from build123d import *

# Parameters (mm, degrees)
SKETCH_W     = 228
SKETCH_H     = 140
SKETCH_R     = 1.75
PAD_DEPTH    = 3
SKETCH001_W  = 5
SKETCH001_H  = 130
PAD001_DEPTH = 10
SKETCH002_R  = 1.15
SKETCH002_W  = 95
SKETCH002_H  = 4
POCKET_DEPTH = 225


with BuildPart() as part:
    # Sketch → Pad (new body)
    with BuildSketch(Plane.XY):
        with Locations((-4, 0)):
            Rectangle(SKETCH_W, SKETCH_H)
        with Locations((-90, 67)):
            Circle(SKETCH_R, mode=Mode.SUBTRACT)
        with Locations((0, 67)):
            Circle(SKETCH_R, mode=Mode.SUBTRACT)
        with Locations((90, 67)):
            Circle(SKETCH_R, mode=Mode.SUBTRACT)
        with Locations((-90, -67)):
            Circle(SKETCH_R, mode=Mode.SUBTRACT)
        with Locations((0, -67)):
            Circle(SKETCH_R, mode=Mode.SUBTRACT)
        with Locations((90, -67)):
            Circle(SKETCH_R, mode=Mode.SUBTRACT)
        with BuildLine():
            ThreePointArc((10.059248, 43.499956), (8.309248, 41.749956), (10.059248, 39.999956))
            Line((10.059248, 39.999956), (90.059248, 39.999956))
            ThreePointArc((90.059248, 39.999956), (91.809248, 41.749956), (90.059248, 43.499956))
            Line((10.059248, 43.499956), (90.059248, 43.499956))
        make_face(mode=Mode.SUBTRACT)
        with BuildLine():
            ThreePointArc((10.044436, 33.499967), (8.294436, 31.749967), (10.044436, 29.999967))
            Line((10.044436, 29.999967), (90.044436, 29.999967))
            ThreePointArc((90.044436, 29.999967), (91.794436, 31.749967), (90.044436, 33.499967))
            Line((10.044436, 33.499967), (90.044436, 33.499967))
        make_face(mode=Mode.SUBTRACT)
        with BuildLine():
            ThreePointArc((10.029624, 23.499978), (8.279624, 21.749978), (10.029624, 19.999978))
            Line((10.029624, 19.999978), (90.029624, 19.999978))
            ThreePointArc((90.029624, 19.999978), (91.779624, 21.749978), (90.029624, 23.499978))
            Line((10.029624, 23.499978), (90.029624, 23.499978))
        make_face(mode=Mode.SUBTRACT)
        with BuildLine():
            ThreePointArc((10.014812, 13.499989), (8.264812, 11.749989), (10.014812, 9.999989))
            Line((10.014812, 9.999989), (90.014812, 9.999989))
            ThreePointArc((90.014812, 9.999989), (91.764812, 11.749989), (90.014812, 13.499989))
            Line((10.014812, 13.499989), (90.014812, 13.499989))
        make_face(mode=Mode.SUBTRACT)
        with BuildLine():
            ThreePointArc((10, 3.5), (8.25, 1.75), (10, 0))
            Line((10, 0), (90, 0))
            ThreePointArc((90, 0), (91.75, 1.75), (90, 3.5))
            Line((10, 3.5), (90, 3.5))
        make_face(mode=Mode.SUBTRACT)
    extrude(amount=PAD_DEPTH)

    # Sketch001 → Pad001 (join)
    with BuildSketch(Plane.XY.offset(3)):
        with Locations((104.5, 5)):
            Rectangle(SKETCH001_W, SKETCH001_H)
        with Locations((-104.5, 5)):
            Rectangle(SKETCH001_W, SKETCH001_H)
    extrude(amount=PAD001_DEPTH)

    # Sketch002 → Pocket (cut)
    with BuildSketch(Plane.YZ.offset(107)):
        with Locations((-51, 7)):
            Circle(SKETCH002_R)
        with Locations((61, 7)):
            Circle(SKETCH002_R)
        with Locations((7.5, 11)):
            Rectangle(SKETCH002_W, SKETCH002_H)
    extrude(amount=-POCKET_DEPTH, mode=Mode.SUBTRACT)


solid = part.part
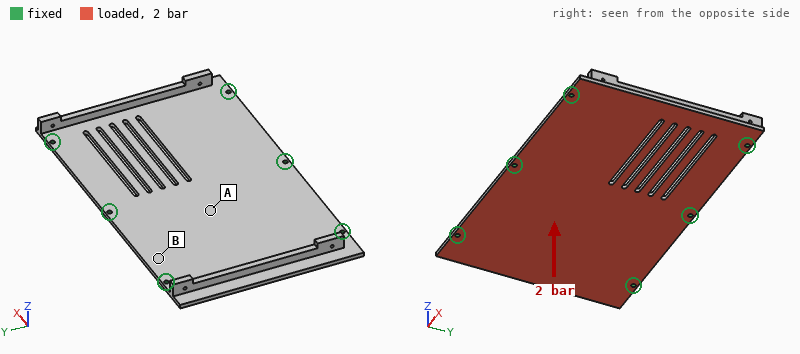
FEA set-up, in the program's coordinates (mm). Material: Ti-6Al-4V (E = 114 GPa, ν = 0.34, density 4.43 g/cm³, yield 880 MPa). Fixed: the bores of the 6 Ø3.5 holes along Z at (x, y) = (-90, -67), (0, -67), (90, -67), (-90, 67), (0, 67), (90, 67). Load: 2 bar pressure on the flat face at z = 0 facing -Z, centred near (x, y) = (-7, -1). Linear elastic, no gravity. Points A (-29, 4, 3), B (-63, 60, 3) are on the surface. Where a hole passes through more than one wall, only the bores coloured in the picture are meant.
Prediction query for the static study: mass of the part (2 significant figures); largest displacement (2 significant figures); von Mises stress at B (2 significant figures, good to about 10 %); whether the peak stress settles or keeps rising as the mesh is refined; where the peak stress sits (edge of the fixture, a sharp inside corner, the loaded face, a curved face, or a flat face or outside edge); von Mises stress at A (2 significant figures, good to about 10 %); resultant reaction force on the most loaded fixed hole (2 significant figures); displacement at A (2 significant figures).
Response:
440 g
1.5 mm
46 MPa
keeps rising
edge of the fixture
120 MPa
1.5 kN
1.1 mm
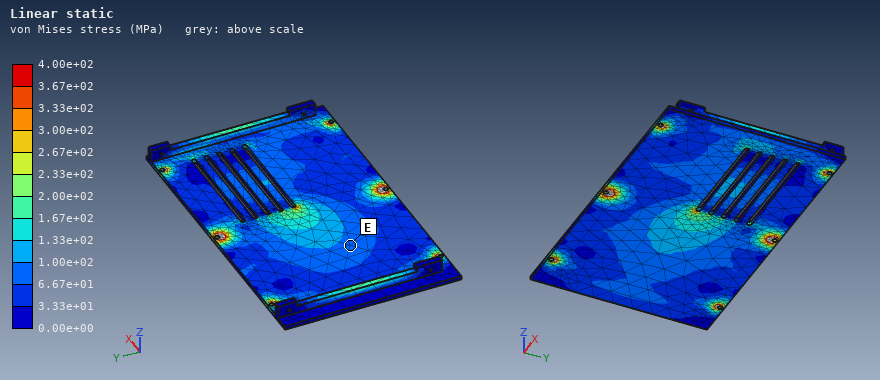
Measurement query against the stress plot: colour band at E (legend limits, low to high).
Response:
6.67e+01 to 1.00e+02 MPa
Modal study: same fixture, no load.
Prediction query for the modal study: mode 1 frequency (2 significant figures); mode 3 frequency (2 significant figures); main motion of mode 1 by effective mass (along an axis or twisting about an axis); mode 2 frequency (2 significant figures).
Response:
670 Hz
1100 Hz
along Z
920 Hz
